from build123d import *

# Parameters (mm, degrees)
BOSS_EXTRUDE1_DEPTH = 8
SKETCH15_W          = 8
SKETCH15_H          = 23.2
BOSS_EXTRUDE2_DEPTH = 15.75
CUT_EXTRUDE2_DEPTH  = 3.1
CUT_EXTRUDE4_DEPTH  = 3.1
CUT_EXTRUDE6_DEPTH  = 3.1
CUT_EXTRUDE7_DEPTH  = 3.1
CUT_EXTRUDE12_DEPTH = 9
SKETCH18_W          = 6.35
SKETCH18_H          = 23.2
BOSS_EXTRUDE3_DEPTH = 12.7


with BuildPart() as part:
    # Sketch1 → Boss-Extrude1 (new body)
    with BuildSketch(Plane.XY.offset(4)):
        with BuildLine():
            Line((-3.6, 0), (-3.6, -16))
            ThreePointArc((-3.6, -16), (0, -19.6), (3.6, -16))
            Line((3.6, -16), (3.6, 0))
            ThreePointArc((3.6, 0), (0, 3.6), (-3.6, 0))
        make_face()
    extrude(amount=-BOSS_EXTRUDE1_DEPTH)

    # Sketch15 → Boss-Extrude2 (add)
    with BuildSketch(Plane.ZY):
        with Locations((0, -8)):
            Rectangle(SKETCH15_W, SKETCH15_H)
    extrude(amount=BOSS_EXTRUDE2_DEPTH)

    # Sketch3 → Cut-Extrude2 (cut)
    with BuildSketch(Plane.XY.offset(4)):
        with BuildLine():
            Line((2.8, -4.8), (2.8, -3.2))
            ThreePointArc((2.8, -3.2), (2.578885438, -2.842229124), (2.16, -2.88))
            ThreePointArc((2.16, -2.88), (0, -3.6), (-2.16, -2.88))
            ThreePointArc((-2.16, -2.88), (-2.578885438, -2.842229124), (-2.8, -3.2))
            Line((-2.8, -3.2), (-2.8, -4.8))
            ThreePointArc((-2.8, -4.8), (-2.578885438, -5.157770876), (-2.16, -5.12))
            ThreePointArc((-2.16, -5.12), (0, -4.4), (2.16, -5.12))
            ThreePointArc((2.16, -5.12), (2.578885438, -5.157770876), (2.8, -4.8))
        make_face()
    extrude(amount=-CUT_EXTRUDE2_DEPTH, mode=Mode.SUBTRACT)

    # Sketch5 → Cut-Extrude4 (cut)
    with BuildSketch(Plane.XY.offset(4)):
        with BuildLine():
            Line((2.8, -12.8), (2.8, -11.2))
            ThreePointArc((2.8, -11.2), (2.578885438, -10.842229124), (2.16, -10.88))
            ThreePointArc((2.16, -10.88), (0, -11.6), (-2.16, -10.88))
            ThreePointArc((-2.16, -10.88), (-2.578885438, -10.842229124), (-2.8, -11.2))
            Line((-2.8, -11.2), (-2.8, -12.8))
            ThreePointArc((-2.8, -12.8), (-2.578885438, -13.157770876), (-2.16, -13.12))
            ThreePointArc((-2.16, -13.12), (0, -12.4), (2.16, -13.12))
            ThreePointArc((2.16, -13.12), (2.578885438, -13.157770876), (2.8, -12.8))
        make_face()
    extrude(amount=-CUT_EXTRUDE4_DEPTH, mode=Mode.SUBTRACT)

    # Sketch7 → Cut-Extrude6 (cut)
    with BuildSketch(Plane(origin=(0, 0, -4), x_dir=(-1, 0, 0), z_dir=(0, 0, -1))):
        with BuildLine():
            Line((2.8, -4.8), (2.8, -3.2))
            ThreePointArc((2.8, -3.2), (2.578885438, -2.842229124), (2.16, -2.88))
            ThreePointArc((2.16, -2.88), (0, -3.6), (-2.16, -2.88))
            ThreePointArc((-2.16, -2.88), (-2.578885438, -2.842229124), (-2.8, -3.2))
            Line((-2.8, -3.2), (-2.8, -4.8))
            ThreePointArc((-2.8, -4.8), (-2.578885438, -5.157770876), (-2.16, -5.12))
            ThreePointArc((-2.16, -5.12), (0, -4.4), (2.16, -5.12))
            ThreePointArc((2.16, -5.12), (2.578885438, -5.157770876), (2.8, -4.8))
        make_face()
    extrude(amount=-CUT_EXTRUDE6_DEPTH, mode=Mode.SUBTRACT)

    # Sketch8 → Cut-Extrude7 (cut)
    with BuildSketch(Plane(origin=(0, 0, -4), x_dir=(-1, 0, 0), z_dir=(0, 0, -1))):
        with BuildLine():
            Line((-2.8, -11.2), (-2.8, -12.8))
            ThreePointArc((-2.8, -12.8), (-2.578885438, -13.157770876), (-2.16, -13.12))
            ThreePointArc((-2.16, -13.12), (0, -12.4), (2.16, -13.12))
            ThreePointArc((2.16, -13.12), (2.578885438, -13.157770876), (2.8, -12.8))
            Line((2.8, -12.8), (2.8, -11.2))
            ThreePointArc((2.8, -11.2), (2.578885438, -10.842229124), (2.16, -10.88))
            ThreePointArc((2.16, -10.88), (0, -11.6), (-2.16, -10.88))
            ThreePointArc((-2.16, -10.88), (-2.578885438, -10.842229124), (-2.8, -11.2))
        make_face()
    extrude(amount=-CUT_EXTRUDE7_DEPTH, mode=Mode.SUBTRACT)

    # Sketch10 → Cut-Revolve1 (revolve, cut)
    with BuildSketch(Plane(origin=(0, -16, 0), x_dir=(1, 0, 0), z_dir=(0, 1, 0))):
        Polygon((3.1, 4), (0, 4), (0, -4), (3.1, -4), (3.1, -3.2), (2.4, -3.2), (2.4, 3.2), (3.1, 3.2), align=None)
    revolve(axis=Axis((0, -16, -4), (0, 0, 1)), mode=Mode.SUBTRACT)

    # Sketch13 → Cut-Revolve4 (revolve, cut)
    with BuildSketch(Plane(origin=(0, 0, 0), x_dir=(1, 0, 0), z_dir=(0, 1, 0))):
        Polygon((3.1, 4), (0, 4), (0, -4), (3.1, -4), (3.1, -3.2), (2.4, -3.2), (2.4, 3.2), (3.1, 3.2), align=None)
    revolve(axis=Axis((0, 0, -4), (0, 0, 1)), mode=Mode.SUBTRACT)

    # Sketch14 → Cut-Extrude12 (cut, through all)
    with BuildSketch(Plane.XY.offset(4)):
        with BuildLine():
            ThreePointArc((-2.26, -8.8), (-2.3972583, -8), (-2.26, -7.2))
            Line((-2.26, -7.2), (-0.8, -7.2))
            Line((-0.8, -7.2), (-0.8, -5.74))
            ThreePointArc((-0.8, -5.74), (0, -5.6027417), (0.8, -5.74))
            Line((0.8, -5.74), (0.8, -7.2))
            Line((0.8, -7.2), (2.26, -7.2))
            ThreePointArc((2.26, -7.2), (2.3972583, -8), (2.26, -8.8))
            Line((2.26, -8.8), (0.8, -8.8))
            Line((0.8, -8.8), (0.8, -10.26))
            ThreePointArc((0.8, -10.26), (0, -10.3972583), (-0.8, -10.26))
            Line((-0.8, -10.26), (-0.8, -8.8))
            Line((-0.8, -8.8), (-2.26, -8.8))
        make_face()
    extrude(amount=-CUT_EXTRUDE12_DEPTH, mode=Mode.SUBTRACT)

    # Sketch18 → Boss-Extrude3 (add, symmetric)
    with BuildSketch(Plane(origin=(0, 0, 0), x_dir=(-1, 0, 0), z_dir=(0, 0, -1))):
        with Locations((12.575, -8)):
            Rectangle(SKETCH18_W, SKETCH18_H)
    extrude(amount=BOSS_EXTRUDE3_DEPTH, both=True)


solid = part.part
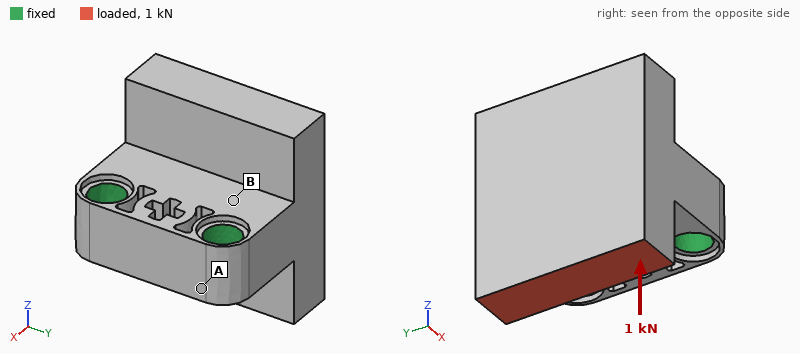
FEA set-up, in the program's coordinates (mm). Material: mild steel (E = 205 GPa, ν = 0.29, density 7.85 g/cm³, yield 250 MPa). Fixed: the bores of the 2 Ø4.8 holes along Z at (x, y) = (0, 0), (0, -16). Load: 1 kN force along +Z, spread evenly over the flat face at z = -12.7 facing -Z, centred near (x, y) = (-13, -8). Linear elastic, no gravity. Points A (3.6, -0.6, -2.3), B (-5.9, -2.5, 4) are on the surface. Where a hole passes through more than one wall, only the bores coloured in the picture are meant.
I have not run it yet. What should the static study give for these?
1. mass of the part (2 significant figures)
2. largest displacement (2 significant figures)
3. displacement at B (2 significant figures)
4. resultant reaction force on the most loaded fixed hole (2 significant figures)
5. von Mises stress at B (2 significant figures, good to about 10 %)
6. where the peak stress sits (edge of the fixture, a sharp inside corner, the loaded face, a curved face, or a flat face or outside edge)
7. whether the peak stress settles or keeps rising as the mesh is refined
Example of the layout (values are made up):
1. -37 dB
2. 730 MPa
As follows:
1. 44 g
2. 10 µm
3. 2.5 µm
4. 500 N
5. 25 MPa
6. edge of the fixture
7. keeps rising
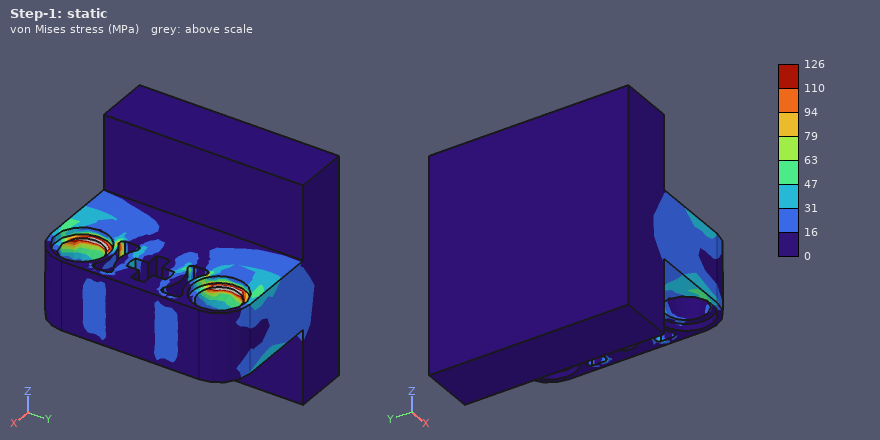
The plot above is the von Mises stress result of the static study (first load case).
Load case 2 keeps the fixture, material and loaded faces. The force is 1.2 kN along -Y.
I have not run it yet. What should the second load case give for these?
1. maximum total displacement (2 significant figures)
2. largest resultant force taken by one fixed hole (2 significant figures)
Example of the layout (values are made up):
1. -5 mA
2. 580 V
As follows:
1. 9.4 µm
2. 1.2 kN
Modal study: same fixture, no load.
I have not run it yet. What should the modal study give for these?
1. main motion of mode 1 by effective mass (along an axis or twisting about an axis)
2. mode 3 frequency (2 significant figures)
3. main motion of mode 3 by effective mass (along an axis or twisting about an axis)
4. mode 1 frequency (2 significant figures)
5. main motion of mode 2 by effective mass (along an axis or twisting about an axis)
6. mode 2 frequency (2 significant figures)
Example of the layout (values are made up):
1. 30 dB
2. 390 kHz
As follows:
1. along Z
2. 24 kHz
3. along Y
4. 9700 Hz
5. twisting about X
6. 18 kHz
